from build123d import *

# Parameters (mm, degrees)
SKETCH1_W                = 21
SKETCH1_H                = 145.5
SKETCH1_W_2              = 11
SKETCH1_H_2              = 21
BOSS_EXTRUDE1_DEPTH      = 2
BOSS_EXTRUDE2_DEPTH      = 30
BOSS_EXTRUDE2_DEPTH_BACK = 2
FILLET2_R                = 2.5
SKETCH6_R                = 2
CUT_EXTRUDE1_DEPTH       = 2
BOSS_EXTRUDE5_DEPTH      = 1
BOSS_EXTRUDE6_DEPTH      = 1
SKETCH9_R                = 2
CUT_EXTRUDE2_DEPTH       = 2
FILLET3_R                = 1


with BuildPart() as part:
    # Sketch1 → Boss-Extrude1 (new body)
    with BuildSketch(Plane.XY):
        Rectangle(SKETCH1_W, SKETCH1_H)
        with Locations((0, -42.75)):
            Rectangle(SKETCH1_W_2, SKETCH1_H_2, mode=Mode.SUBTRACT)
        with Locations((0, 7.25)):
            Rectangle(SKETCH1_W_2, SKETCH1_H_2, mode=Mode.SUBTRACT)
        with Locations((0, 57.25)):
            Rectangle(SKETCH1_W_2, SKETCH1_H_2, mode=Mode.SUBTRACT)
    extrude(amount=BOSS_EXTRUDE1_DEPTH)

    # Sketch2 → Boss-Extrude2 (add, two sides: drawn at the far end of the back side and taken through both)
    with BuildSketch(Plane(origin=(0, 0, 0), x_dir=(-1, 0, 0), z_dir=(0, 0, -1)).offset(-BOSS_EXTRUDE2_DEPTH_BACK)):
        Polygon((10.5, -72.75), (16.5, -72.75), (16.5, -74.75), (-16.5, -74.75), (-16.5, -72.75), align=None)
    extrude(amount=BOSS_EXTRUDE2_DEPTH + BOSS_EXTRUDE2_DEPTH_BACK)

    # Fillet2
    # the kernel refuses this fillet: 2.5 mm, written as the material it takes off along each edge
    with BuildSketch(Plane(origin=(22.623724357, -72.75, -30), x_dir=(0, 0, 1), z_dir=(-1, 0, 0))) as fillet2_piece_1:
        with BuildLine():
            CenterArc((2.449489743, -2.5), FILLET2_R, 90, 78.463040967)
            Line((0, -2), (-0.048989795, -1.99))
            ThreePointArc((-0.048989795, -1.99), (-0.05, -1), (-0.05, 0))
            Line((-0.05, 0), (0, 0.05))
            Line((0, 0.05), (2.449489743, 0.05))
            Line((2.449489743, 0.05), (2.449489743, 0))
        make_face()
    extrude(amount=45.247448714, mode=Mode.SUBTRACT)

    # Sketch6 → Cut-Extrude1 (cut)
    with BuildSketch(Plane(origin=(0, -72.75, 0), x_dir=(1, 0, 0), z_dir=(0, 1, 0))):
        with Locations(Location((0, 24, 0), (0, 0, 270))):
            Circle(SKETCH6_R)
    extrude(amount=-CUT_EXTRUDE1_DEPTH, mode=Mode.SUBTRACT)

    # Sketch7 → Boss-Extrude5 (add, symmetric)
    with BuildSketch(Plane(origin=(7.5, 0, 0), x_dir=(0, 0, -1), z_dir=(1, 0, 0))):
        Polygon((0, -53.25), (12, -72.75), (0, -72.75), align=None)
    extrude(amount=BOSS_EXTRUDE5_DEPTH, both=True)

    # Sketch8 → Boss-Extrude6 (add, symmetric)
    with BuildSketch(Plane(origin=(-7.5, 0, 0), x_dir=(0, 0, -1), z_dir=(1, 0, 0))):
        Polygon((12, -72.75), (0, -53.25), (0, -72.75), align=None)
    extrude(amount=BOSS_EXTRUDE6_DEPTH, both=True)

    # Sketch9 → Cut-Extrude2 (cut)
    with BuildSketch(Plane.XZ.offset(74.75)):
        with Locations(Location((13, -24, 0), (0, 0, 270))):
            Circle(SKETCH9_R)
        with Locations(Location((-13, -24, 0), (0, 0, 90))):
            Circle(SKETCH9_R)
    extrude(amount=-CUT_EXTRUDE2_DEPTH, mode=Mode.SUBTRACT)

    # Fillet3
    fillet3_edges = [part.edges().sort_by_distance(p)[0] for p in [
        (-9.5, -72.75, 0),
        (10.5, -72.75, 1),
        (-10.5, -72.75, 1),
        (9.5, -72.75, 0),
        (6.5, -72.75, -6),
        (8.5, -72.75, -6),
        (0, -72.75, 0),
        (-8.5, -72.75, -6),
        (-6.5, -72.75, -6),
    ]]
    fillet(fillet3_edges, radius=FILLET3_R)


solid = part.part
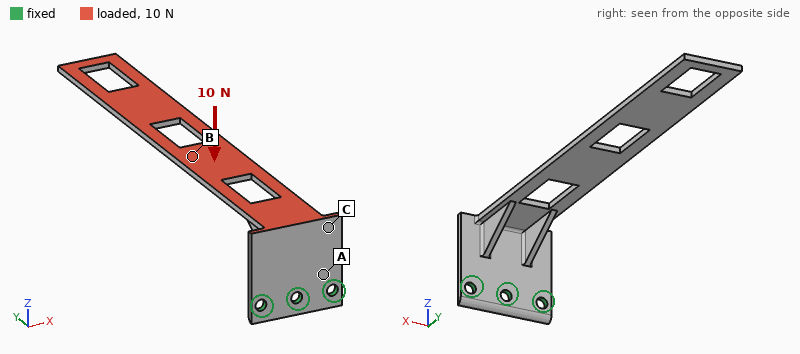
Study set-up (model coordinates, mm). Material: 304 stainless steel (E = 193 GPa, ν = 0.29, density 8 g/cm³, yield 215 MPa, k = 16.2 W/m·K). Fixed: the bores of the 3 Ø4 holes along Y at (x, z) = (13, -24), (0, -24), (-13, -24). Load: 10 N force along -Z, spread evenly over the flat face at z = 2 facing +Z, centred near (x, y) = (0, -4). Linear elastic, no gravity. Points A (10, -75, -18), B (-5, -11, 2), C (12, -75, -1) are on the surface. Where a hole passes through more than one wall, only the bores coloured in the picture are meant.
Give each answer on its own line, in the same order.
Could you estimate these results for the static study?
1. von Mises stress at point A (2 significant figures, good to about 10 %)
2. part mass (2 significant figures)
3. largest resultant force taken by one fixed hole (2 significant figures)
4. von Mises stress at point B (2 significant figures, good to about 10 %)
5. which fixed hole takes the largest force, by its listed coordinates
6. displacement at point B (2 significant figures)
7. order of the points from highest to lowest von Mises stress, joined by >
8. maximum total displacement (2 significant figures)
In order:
27 MPa
58 g
8.7 N
16 MPa
(0, -24)
0.44 mm
A > B > C
1.8 mm
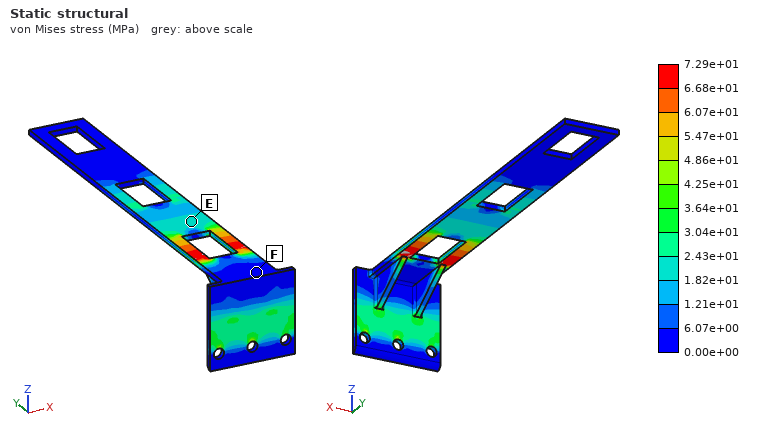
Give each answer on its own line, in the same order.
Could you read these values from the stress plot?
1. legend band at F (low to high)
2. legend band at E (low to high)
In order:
0.00e+00 to 6.07e+00 MPa
1.82e+01 to 2.43e+01 MPa
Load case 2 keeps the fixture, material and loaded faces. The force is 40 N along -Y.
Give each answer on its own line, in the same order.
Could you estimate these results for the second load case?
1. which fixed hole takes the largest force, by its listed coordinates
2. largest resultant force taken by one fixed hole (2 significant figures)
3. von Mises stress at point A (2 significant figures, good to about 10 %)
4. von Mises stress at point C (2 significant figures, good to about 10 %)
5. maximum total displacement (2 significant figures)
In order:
(0, -24)
21 N
32 MPa
4.6 MPa
0.45 mm
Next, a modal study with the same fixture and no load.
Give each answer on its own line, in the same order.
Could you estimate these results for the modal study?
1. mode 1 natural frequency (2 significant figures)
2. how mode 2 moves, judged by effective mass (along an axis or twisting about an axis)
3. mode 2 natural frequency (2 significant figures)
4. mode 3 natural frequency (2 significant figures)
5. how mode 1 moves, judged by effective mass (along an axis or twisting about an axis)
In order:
77 Hz
along X
270 Hz
440 Hz
along Z
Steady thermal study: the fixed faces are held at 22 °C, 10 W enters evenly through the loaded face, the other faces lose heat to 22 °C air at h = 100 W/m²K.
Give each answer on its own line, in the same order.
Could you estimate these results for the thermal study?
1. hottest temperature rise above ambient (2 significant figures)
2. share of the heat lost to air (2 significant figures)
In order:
31 K
97 %
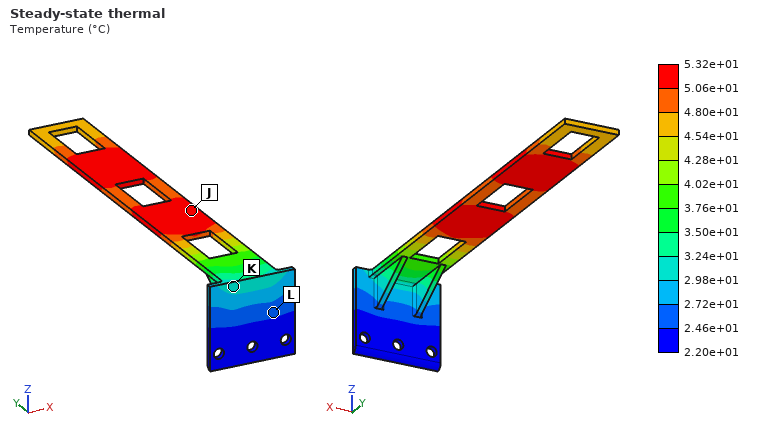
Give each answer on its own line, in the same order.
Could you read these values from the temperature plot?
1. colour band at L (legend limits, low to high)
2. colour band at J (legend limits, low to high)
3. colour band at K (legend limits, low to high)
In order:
2.46e+01 to 2.72e+01 °C
5.06e+01 to 5.32e+01 °C
2.98e+01 to 3.24e+01 °C
